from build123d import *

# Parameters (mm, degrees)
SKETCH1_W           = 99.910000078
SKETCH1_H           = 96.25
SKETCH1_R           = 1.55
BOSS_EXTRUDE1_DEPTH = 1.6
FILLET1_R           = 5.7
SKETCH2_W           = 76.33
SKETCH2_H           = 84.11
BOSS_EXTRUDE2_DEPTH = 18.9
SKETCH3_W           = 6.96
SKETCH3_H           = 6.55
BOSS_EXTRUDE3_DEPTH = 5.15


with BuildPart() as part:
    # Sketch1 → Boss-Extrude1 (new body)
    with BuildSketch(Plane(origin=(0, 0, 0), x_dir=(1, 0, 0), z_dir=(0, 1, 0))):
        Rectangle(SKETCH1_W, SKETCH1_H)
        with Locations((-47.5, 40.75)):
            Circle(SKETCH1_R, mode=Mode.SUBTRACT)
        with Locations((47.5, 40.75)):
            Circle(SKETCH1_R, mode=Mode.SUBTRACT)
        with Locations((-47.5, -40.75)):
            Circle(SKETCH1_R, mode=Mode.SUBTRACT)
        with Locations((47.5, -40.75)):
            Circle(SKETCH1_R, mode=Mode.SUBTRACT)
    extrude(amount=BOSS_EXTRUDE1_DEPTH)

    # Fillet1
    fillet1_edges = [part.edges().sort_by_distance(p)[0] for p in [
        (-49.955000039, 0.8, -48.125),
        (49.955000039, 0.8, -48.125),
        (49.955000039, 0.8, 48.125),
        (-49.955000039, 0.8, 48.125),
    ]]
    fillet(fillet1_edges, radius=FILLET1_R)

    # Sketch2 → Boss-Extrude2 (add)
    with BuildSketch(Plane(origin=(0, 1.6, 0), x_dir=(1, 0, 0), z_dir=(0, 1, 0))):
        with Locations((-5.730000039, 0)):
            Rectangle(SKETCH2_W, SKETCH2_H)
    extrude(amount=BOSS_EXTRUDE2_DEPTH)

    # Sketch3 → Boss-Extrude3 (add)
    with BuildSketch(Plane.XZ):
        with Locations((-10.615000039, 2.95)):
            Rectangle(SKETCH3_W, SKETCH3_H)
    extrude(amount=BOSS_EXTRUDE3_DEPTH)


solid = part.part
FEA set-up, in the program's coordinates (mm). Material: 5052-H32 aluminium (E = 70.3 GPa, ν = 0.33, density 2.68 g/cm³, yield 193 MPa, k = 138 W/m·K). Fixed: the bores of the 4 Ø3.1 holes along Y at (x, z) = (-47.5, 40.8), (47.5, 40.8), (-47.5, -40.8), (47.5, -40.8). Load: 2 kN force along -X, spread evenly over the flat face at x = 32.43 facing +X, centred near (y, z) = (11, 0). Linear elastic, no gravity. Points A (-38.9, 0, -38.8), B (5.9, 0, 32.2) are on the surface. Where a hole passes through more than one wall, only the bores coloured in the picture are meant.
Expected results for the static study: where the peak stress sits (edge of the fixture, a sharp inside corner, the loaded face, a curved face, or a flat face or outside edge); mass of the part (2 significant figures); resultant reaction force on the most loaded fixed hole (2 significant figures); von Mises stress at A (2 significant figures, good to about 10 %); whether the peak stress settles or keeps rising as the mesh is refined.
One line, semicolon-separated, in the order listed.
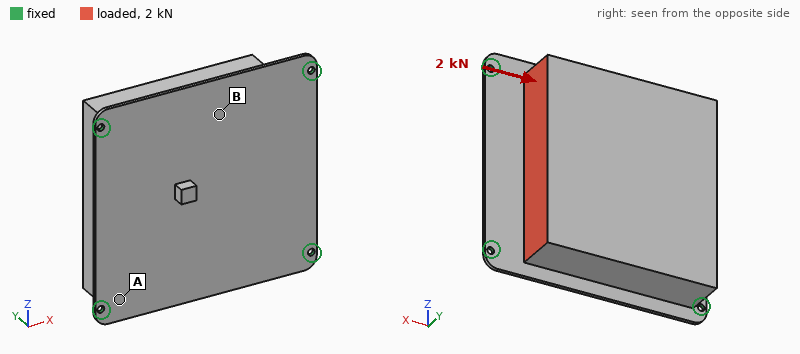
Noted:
edge of the fixture; 370 g; 600 N; 13 MPa; keeps rising
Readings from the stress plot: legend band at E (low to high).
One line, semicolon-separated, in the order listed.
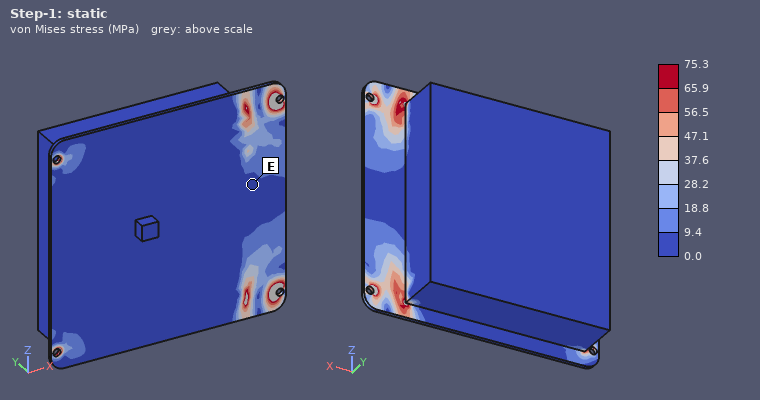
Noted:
0.0 to 9.4 MPa
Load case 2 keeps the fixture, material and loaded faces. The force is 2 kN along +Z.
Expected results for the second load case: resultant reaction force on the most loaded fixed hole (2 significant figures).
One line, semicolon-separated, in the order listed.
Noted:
760 N
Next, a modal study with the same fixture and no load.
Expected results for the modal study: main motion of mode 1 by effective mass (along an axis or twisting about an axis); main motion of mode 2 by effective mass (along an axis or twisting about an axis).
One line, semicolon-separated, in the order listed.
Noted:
along Y; along Z
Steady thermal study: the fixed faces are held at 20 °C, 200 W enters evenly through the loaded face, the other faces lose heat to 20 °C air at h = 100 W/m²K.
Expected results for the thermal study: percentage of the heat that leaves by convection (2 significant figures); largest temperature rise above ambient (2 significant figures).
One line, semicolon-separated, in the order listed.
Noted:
65 %; 79 K
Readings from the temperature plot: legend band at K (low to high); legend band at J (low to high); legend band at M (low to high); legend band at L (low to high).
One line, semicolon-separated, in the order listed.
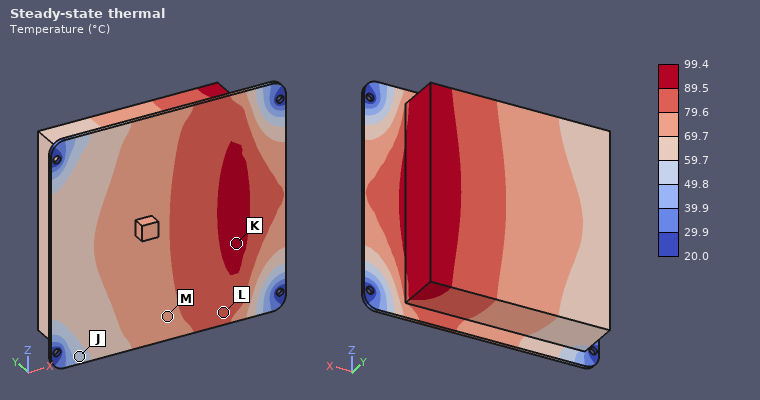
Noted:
89.5 to 99.4 °C; 49.8 to 59.7 °C; 69.7 to 79.6 °C; 79.6 to 89.5 °C
